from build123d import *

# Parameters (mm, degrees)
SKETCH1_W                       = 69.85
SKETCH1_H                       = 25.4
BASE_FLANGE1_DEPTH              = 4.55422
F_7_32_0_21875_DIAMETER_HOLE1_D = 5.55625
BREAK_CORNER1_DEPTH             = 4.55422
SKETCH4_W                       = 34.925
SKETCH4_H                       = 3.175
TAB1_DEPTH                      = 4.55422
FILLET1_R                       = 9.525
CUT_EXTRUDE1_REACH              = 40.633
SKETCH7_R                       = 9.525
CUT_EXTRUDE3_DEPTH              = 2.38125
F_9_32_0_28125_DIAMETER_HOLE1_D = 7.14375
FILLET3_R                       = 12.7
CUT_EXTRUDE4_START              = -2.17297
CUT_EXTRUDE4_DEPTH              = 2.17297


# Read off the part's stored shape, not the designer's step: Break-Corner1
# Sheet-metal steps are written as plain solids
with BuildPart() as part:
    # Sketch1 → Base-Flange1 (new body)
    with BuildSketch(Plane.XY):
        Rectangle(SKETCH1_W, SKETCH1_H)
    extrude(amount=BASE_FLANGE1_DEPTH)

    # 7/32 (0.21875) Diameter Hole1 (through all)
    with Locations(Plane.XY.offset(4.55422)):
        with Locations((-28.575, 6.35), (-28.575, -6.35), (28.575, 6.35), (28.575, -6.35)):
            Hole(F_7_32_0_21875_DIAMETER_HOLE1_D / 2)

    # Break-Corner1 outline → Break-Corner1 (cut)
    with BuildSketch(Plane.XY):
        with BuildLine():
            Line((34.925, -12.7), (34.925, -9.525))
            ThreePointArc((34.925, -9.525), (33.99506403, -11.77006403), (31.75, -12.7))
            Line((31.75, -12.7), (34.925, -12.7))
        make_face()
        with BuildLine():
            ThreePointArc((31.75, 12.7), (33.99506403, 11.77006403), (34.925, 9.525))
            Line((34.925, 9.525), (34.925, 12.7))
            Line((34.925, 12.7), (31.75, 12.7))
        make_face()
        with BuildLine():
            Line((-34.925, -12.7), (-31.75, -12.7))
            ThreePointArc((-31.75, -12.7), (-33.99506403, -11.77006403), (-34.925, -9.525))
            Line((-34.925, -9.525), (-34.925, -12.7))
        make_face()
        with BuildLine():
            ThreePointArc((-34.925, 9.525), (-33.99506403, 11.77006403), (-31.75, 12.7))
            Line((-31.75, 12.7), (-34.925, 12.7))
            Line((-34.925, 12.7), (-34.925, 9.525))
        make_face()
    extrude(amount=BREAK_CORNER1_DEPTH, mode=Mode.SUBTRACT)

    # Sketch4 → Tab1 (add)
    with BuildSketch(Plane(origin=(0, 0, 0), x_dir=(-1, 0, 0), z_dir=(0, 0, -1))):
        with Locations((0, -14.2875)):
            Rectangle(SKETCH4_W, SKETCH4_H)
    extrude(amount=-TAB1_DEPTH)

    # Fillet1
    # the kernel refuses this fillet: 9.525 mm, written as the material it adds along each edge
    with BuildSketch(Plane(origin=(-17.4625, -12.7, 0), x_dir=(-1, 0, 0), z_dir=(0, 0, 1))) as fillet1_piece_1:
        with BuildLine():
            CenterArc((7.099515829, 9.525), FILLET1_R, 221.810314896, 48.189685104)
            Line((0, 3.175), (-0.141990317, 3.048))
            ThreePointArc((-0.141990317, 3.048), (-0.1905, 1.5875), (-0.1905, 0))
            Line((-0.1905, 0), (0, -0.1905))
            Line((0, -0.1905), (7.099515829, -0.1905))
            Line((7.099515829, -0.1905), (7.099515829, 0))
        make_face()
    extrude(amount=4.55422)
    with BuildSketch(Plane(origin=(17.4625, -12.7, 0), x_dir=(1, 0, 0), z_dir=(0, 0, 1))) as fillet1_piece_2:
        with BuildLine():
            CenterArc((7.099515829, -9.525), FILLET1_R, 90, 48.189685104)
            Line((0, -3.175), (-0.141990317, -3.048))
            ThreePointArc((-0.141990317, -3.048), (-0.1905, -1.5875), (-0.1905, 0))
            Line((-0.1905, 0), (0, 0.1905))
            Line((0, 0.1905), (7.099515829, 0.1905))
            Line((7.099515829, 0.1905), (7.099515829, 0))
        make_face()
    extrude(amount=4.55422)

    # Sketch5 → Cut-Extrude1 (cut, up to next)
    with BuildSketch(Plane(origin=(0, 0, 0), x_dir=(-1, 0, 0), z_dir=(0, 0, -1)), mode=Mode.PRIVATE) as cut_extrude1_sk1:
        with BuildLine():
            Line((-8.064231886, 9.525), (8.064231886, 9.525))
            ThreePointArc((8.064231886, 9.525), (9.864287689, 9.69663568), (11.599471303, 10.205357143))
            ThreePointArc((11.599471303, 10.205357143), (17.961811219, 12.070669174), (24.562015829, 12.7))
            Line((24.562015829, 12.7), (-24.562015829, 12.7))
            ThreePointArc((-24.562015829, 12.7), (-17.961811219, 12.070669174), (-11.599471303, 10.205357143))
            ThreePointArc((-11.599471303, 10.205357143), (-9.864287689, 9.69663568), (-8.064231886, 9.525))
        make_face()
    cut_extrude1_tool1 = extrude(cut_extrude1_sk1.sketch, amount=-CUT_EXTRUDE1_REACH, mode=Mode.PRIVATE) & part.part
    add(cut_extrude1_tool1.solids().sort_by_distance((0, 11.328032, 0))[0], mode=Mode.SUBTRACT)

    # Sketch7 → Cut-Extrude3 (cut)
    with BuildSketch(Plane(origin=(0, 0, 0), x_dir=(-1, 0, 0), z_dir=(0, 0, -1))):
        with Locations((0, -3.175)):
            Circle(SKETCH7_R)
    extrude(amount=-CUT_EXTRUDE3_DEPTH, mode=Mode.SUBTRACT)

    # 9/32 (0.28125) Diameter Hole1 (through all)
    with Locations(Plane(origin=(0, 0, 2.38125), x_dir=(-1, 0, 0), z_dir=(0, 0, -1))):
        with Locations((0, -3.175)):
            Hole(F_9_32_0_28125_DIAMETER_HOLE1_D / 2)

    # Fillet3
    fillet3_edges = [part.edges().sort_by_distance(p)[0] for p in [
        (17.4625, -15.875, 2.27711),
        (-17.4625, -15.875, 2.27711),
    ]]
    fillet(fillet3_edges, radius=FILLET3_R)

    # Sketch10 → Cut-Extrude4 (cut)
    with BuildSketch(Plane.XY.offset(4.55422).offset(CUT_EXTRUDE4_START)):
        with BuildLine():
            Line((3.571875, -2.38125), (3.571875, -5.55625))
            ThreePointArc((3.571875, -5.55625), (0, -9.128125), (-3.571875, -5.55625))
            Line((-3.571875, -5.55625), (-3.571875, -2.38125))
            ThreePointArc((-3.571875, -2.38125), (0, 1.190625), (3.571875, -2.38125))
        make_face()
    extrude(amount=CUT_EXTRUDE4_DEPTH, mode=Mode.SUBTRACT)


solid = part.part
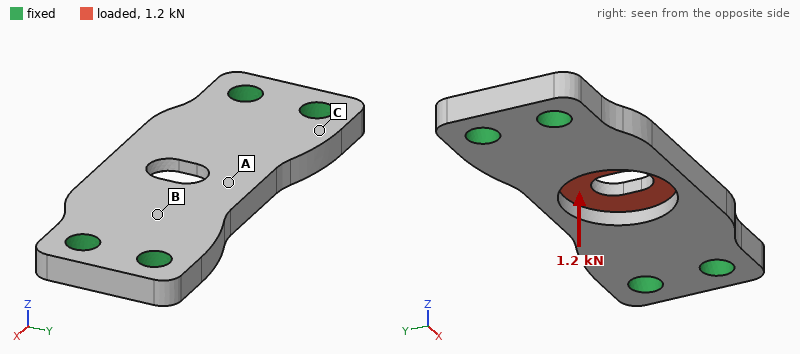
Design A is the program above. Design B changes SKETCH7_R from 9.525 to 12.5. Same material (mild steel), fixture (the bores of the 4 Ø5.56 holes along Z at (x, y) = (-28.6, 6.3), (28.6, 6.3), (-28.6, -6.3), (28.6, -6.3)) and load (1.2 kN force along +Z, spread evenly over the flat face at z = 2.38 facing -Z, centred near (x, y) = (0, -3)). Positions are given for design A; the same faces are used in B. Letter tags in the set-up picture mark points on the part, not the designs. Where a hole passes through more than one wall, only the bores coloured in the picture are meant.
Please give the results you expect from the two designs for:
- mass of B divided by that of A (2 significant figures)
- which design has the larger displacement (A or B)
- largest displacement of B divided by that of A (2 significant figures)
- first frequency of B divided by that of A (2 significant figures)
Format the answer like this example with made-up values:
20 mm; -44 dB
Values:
0.93; B; 1.2; 1.0
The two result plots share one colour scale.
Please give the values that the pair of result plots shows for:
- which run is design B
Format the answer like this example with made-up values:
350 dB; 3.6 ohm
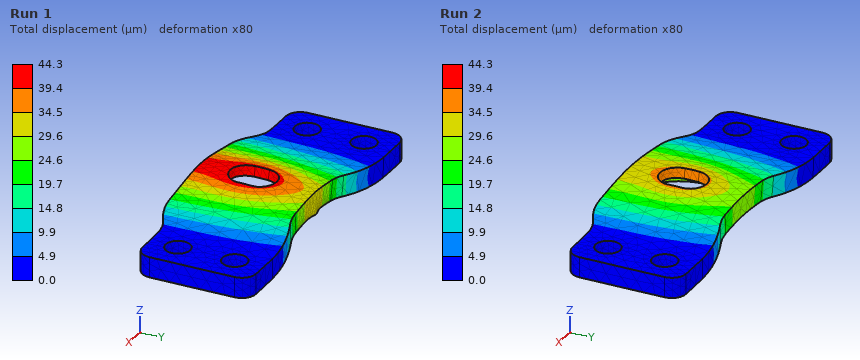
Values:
Run 1
